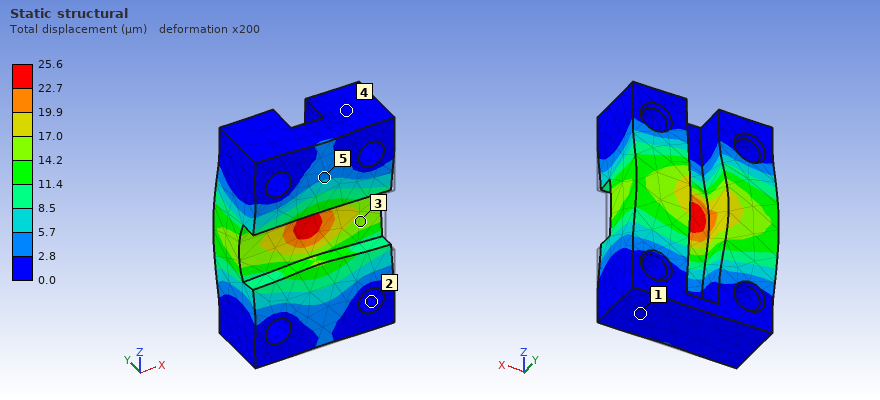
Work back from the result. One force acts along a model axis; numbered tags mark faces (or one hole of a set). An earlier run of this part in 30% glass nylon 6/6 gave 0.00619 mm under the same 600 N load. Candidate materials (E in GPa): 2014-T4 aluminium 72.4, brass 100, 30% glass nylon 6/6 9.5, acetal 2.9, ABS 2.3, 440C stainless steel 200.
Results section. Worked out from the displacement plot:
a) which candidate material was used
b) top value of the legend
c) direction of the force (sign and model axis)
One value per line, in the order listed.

ABS
25.6 µm
+Y
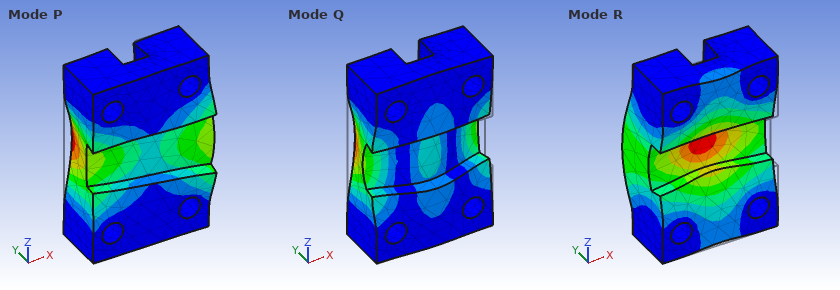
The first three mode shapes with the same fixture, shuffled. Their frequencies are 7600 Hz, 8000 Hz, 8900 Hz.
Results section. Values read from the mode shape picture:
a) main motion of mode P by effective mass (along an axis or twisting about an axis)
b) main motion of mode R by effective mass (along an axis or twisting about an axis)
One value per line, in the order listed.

along X
along Y
